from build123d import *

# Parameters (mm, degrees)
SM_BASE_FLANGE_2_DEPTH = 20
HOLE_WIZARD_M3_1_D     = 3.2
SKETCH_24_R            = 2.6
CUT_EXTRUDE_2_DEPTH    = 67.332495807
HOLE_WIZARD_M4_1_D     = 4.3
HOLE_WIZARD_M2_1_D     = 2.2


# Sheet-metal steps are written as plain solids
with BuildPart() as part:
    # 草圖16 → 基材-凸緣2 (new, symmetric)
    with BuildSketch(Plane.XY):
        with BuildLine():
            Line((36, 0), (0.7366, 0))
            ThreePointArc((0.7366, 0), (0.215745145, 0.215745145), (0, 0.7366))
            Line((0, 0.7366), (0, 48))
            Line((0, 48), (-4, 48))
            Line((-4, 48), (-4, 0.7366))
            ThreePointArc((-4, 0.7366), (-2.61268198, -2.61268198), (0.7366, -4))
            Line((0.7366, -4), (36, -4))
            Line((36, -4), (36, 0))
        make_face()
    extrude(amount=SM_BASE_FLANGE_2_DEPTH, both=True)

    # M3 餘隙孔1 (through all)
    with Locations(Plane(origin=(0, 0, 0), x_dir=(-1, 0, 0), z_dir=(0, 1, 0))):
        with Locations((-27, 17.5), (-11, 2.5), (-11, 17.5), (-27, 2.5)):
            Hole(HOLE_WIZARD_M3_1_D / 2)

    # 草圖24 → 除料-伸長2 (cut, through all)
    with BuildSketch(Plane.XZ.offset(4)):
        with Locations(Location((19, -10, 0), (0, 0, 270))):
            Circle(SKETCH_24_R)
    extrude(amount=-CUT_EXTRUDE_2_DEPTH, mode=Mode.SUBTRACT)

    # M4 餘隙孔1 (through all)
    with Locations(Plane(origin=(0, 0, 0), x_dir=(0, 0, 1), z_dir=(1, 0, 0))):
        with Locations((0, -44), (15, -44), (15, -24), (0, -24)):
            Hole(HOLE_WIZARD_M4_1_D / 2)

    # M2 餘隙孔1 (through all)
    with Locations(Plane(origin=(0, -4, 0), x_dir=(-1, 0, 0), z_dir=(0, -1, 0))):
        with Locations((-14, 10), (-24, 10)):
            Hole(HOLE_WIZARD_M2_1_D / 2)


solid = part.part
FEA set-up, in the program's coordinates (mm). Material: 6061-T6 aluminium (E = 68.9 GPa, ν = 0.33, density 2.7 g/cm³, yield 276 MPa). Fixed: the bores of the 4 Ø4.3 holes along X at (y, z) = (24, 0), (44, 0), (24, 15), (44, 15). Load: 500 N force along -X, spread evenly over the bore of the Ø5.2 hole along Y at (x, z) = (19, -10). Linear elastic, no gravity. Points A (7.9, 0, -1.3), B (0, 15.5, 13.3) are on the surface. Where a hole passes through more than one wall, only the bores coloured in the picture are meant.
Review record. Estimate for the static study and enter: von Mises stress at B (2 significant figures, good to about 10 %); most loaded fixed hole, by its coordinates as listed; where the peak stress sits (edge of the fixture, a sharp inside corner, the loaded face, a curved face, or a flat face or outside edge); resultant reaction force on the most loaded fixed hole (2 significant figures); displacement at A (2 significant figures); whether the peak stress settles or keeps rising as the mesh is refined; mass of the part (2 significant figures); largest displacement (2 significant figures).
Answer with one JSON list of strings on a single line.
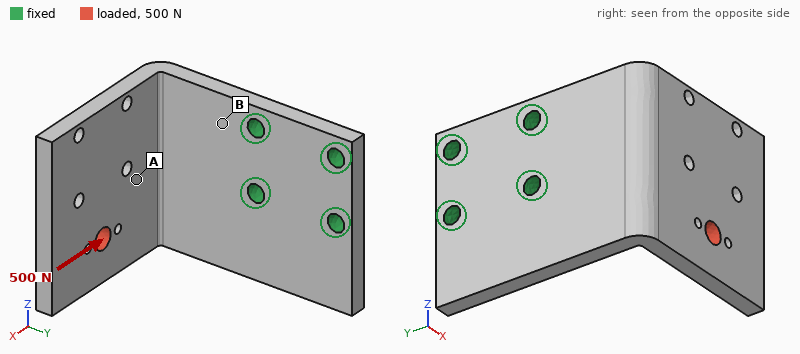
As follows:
["77 MPa", "(24, 0)", "edge of the fixture", "830 N", "0.24 mm", "keeps rising", "36 g", "0.61 mm"]
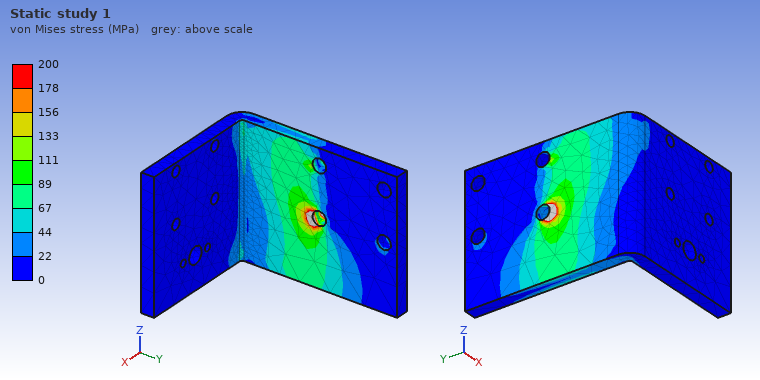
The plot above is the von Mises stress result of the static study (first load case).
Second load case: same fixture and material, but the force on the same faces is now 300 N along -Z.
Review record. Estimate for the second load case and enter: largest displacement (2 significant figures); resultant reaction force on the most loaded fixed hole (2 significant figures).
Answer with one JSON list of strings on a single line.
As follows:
["0.23 mm", "470 N"]
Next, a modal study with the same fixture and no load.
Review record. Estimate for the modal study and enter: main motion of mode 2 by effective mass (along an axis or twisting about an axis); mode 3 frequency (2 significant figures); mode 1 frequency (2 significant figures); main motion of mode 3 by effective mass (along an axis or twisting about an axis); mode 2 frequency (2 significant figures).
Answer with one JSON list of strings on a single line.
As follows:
["along Z", "3100 Hz", "1100 Hz", "along X", "1800 Hz"]
